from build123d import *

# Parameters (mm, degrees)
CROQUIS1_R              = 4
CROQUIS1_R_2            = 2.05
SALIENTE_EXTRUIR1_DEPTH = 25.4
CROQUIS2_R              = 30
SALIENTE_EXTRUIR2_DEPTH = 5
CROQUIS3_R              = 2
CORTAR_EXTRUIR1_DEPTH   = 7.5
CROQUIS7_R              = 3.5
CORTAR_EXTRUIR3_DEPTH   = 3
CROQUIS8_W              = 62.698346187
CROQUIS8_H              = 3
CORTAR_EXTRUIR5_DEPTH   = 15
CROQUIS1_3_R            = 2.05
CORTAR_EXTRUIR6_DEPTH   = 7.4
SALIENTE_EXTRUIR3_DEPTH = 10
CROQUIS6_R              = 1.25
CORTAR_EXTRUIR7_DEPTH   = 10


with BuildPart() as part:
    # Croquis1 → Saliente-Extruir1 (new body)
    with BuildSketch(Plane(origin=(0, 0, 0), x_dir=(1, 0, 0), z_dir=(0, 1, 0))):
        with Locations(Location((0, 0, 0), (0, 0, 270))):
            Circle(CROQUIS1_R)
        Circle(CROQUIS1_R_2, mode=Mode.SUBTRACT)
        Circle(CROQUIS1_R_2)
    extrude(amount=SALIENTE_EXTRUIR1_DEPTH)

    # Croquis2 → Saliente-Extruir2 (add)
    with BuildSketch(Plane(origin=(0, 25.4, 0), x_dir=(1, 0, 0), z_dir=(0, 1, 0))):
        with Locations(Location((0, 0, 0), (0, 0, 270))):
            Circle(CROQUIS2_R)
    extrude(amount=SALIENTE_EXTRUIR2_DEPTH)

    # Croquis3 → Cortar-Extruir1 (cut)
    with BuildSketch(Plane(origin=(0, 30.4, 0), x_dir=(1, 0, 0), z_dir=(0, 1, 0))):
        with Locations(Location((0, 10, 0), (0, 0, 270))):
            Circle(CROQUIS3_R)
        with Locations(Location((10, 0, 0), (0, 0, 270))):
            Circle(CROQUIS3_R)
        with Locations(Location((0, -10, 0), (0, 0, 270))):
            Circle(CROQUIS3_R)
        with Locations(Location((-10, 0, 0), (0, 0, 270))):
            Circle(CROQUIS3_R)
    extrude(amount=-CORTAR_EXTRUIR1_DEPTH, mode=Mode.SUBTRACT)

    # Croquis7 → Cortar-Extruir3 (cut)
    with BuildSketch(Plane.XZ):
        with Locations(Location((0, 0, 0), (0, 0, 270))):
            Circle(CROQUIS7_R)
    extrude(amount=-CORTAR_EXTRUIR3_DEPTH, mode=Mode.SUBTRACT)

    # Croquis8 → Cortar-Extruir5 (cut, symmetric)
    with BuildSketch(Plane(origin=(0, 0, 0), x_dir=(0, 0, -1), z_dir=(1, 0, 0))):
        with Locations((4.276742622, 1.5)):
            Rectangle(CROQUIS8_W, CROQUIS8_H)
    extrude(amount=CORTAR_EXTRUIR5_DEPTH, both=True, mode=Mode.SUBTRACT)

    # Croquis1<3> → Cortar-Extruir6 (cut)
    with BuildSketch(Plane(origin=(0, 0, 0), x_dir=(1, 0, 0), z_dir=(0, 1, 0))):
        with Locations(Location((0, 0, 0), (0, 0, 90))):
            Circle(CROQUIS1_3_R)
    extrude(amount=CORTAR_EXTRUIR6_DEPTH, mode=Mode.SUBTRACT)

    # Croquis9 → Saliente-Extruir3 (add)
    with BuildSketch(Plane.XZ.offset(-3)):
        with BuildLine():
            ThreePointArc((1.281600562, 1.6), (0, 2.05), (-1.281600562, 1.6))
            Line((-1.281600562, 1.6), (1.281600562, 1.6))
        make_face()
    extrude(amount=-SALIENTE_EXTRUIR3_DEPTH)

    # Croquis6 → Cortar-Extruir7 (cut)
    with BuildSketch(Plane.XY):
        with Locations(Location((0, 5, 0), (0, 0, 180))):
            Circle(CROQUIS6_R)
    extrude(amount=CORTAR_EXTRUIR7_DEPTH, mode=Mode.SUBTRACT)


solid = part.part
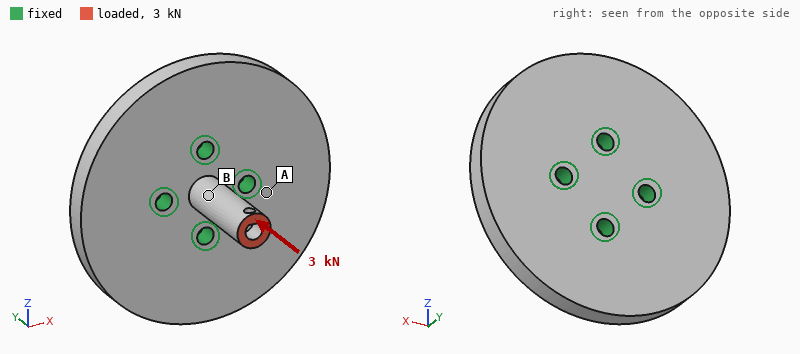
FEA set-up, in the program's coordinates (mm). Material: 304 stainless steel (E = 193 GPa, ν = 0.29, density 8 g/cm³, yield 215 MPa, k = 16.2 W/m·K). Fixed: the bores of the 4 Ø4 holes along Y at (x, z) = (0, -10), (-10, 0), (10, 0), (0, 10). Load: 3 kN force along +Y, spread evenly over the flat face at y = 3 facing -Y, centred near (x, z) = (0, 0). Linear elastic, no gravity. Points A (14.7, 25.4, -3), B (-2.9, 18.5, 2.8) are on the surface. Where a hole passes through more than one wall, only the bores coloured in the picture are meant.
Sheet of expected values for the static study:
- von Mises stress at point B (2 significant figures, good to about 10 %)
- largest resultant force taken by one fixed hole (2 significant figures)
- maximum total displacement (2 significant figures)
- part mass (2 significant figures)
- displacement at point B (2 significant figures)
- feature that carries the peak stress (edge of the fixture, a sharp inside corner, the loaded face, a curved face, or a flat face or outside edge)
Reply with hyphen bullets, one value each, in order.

- 61 MPa
- 780 N
- 15 µm
- 120 g
- 4.9 µm
- a curved face
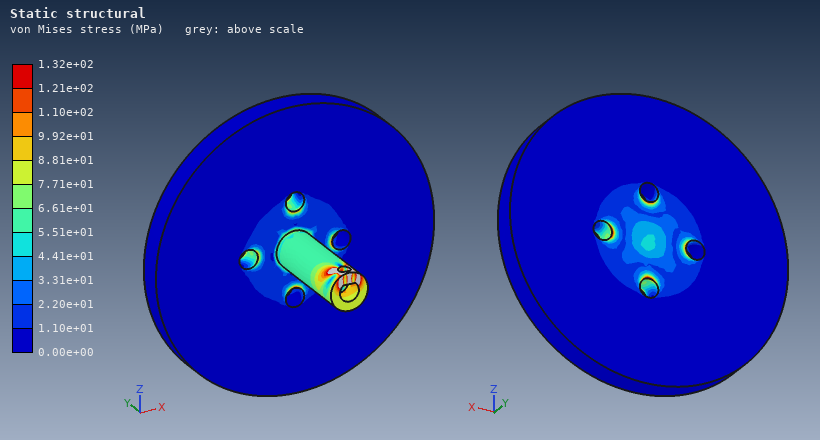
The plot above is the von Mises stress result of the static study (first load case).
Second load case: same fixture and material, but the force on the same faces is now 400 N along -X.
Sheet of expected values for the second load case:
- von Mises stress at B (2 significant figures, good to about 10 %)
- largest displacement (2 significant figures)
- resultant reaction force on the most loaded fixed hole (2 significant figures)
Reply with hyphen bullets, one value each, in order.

- 89 MPa
- 57 µm
- 600 N
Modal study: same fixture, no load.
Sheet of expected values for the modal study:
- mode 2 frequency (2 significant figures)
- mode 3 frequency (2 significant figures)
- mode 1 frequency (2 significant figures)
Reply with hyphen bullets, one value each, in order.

- 8600 Hz
- 8900 Hz
- 8600 Hz
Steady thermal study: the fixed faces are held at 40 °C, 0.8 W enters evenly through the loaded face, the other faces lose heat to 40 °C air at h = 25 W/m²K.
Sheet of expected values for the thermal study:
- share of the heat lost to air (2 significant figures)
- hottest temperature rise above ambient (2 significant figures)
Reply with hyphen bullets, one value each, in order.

- 27 %
- 25 K
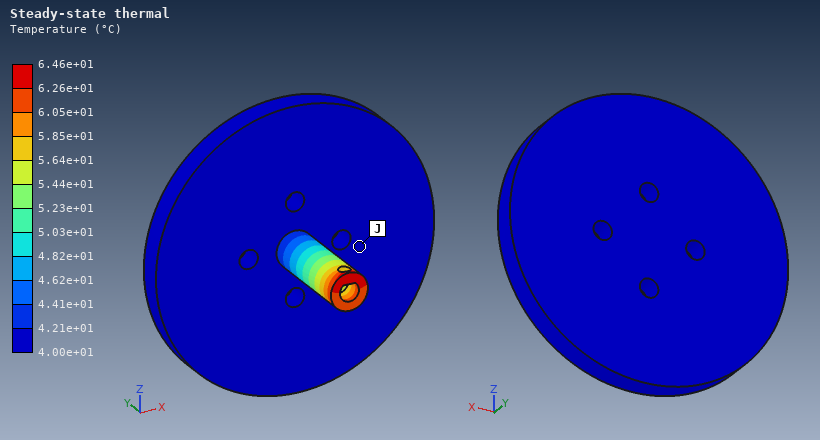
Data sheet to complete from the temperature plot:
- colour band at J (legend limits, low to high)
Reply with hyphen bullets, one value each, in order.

- 4.00e+01 to 4.21e+01 °C
